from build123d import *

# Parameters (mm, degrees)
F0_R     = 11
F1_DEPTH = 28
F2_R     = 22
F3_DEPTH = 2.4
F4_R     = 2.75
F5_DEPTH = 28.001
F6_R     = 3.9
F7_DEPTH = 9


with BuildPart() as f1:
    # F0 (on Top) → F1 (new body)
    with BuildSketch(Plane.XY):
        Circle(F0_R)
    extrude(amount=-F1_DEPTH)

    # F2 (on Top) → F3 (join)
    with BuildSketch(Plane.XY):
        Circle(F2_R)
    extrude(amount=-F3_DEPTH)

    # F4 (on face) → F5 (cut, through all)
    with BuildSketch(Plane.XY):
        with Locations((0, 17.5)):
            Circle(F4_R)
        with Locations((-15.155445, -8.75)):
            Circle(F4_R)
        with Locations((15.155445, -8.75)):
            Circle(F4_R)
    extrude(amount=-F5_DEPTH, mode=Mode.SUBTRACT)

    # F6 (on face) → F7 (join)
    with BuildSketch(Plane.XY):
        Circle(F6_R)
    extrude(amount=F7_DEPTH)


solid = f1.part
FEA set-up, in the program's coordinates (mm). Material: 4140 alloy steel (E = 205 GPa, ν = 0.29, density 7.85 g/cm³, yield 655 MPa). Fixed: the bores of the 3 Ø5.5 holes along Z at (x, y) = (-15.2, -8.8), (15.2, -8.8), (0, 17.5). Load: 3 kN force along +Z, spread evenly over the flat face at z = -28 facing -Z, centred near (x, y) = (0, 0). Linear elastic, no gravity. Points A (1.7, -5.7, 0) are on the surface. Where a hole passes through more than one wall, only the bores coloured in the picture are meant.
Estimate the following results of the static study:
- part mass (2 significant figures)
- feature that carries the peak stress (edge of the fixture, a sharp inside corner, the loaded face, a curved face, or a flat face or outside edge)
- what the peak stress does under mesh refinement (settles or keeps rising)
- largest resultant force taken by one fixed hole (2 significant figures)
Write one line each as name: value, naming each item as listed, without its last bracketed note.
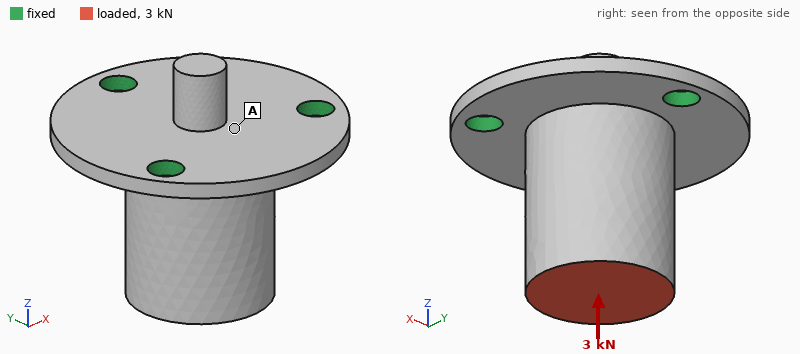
part mass: 110 g
feature that carries the peak stress: edge of the fixture
what the peak stress does under mesh refinement: keeps rising
largest resultant force taken by one fixed hole: 1.1 kN
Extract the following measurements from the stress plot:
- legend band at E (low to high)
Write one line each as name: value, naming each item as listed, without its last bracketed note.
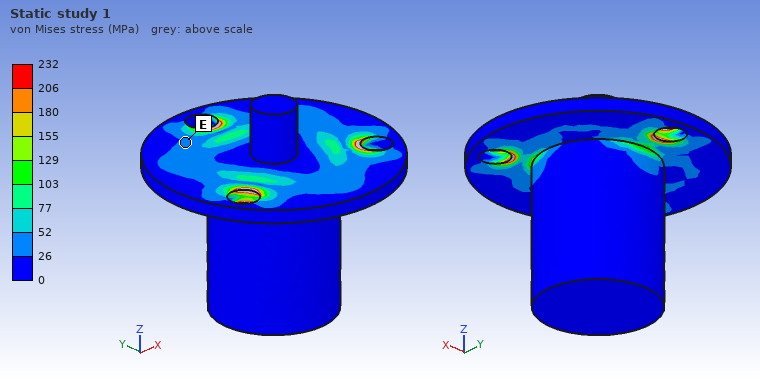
legend band at E: 26 to 52 MPa
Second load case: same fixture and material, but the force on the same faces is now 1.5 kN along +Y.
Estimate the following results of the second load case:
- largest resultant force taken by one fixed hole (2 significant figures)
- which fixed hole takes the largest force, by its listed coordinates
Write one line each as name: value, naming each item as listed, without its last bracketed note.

largest resultant force taken by one fixed hole: 2.0 kN
which fixed hole takes the largest force, by its listed coordinates: (0, 17.5)
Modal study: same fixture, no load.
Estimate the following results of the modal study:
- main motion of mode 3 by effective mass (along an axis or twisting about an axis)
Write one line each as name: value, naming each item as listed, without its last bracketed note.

main motion of mode 3 by effective mass: along Z
